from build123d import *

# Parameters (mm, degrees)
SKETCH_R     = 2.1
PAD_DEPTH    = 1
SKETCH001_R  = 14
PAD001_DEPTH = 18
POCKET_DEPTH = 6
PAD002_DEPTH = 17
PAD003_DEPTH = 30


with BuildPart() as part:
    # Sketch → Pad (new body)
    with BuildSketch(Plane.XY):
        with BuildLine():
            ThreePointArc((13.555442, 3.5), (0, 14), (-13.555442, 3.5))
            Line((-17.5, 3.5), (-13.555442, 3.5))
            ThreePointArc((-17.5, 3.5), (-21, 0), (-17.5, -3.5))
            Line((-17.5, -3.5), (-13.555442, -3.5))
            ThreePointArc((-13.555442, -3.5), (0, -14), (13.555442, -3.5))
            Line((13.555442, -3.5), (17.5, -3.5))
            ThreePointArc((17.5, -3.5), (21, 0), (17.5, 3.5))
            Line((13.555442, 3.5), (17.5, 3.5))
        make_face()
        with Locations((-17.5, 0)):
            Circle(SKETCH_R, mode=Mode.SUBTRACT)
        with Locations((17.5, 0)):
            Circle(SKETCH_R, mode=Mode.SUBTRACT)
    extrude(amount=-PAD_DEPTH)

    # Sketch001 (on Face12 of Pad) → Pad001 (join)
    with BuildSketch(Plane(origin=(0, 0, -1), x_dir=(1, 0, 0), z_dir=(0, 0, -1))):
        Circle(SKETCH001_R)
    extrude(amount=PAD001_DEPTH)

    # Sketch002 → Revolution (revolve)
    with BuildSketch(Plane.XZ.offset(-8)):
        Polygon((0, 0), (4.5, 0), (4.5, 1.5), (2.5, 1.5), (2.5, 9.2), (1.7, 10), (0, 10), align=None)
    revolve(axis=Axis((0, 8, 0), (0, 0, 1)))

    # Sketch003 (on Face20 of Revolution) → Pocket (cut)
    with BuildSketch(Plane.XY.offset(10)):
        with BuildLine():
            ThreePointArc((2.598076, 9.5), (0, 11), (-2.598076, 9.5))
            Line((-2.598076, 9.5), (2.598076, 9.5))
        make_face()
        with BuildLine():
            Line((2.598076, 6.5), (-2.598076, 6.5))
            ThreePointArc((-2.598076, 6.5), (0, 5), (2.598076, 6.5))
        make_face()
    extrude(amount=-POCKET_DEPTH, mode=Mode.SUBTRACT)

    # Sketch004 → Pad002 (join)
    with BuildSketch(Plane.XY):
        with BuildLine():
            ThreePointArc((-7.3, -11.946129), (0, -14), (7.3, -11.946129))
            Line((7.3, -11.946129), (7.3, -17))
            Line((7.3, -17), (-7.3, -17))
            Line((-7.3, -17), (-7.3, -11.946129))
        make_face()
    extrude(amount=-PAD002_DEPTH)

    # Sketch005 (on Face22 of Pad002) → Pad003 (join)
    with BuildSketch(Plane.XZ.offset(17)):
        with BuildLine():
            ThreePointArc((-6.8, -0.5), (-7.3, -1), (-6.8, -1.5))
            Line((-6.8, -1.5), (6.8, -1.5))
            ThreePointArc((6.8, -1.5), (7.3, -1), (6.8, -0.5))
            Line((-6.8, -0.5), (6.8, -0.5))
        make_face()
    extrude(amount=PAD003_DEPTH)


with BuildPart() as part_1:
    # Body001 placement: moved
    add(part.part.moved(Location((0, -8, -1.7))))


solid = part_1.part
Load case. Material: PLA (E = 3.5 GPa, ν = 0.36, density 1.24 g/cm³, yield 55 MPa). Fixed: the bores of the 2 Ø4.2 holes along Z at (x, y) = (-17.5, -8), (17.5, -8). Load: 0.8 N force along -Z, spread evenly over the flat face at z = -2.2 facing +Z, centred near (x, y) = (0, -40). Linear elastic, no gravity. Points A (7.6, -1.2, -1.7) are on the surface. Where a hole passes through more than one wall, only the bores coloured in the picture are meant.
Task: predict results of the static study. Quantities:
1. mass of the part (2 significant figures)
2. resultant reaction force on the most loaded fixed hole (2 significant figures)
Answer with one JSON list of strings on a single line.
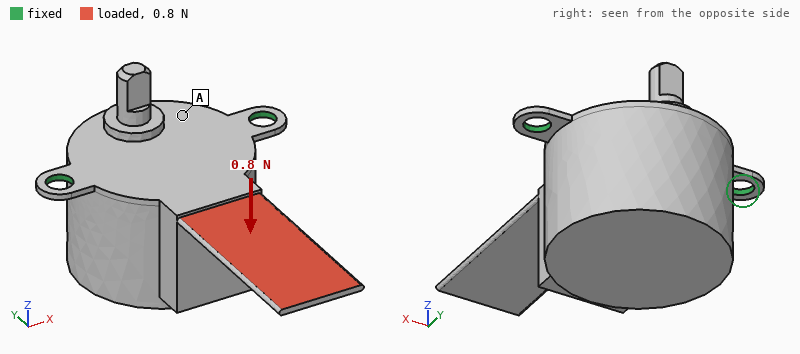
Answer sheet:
["17 g", "0.50 N"]
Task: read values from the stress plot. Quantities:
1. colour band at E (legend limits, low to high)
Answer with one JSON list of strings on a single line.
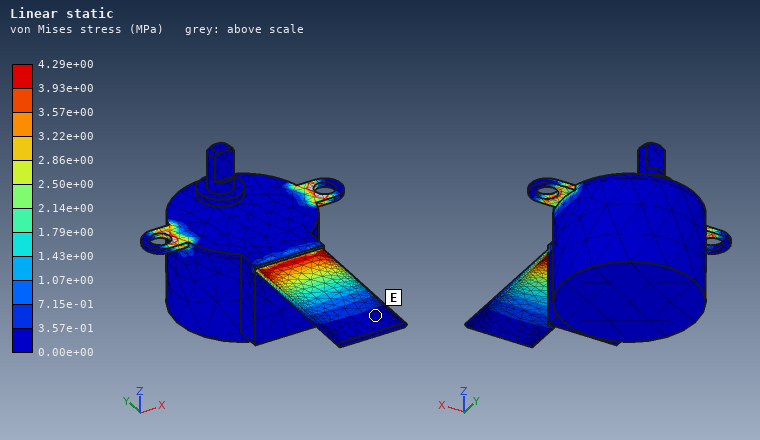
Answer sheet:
["0.00e+00 to 3.57e-01 MPa"]
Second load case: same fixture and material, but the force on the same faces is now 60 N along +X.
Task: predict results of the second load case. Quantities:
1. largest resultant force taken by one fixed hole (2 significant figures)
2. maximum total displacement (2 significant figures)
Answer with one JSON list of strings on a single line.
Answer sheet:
["69 N", "0.67 mm"]
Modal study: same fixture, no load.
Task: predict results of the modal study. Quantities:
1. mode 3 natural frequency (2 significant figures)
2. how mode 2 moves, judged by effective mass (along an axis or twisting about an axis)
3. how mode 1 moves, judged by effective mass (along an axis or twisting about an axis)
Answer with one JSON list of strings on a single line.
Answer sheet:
["1300 Hz", "along Y", "along Y"]
